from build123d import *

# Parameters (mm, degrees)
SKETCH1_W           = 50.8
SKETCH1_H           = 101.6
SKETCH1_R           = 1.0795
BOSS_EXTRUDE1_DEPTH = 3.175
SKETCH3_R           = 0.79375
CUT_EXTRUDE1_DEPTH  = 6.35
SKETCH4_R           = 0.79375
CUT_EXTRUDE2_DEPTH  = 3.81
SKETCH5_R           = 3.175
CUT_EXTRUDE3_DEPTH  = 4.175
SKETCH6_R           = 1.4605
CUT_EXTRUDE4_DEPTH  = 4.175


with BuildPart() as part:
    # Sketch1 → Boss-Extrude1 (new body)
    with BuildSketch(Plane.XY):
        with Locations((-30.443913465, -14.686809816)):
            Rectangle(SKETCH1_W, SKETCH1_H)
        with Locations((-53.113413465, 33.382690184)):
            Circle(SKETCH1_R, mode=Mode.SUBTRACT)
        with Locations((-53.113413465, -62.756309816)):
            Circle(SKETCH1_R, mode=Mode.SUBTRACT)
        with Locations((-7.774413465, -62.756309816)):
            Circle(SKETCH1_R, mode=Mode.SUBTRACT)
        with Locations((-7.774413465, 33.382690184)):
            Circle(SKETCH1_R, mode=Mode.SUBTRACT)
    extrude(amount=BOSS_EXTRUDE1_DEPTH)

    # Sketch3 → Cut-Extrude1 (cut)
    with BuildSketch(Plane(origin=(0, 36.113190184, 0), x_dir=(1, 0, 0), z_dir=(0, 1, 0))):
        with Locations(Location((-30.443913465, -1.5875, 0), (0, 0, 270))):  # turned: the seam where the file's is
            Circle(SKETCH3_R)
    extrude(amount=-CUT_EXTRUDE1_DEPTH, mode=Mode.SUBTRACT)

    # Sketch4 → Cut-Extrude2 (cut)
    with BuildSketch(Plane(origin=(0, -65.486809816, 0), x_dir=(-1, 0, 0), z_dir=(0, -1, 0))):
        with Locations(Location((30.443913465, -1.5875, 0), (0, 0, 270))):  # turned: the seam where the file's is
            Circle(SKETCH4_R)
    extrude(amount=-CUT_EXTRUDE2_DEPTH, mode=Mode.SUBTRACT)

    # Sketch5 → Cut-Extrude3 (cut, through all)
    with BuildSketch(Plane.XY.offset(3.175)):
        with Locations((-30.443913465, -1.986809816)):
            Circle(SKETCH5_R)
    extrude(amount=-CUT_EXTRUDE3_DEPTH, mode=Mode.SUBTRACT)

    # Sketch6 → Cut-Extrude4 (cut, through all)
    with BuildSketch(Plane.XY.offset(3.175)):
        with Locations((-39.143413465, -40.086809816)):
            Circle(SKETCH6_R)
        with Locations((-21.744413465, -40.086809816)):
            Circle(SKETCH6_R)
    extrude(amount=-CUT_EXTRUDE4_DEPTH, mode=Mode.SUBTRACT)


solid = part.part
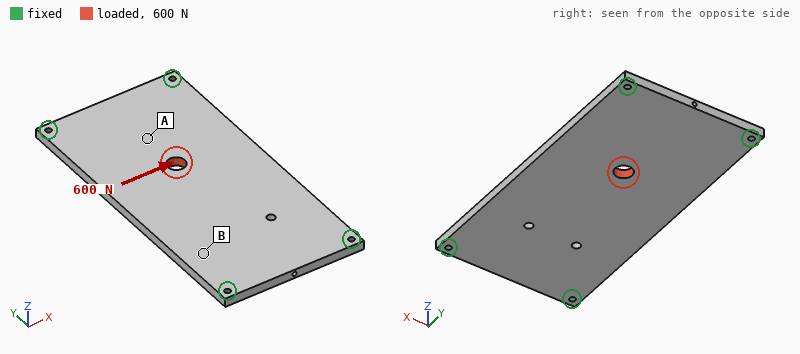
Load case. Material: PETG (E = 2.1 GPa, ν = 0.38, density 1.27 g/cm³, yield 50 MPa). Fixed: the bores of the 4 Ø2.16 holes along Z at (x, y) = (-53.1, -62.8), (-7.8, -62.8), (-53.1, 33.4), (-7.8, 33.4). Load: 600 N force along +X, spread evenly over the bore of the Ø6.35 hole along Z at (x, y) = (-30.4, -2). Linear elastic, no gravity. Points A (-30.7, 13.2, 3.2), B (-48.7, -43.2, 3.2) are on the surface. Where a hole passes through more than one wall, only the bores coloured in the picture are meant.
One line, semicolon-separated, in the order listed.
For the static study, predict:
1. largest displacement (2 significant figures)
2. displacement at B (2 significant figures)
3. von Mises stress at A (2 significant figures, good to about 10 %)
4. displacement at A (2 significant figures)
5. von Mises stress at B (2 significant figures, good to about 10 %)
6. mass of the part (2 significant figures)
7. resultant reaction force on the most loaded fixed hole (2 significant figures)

0.20 mm; 0.067 mm; 5.6 MPa; 0.11 mm; 2.2 MPa; 21 g; 260 N
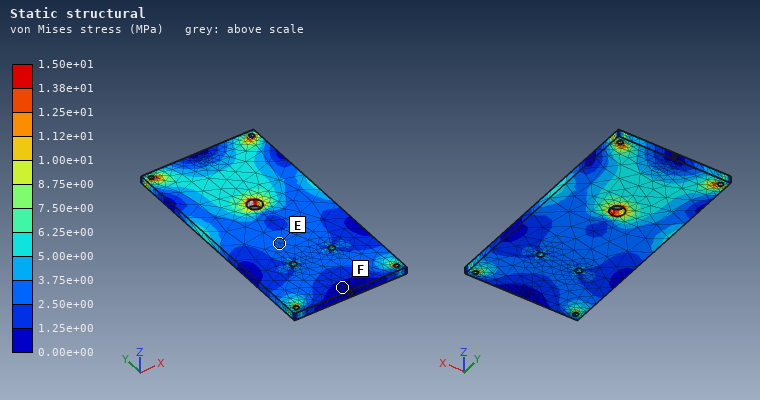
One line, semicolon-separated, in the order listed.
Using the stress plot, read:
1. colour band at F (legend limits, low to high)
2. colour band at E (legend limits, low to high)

0.00e+00 to 1.25e+00 MPa; 2.50e+00 to 3.75e+00 MPa
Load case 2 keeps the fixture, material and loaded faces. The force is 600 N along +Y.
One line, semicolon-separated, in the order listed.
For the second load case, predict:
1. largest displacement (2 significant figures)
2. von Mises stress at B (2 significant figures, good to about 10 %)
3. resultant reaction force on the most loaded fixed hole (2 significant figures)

0.10 mm; 2.2 MPa; 190 N
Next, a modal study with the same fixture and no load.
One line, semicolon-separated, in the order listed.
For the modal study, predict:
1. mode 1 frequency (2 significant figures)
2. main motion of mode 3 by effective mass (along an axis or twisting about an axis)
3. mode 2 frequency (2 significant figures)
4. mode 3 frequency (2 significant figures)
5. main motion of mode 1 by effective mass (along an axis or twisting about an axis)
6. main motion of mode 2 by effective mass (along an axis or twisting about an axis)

360 Hz; twisting about X; 680 Hz; 1000 Hz; along Z; twisting about Y
